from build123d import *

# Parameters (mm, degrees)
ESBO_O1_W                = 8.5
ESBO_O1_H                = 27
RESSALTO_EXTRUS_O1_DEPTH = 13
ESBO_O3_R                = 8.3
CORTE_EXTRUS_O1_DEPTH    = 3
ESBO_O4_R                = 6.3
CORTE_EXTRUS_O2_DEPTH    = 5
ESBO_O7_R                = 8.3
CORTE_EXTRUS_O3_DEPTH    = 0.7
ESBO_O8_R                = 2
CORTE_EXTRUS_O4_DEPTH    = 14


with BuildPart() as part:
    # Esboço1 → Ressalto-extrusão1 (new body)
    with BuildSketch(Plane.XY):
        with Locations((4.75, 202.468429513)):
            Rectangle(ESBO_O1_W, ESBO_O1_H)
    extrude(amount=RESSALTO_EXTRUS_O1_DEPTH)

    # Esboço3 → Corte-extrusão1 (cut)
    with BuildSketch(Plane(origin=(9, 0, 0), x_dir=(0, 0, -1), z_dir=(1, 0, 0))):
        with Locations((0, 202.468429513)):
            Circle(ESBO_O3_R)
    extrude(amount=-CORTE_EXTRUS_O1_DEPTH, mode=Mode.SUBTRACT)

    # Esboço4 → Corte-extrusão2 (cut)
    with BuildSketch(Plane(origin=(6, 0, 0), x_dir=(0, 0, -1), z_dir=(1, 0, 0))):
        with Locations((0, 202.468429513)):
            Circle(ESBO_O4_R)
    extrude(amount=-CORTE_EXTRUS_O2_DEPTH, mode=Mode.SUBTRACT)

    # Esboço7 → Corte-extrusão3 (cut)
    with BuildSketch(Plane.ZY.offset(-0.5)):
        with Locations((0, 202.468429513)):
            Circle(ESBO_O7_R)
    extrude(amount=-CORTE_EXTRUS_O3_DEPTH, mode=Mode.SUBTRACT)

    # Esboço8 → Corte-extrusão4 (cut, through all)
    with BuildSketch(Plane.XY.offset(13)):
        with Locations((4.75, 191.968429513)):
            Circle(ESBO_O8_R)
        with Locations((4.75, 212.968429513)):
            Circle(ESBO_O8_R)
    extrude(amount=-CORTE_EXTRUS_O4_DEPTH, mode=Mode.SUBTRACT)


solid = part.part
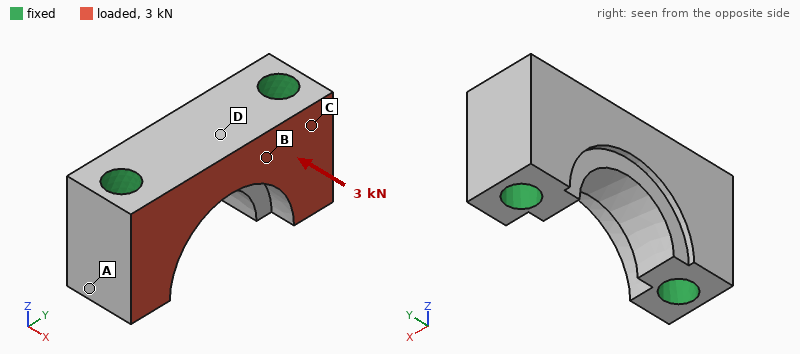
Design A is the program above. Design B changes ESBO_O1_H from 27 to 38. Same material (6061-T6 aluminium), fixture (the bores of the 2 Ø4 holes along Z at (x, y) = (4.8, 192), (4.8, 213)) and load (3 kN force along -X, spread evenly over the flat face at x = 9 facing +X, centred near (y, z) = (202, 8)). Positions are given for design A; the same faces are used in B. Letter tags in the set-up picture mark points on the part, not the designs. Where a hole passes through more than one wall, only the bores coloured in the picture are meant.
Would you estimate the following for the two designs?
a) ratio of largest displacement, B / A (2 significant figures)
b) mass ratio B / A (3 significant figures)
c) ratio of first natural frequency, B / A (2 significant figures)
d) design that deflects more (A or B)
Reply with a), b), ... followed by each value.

a) 0.69
b) 1.62
c) 0.91
d) A
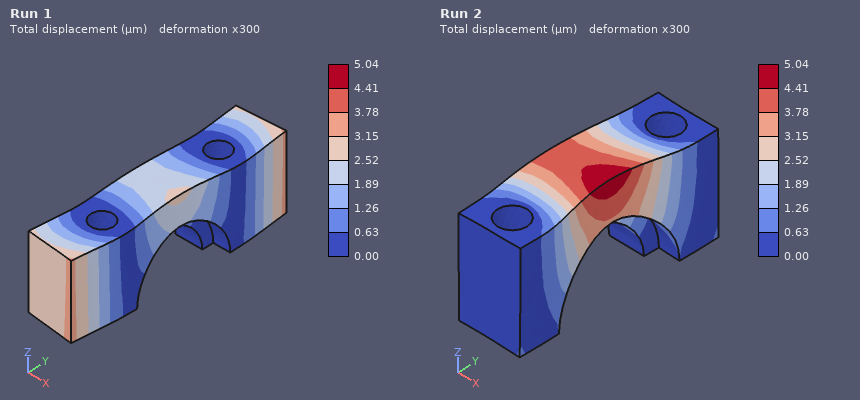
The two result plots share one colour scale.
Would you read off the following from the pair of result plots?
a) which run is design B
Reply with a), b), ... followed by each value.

a) Run 1
